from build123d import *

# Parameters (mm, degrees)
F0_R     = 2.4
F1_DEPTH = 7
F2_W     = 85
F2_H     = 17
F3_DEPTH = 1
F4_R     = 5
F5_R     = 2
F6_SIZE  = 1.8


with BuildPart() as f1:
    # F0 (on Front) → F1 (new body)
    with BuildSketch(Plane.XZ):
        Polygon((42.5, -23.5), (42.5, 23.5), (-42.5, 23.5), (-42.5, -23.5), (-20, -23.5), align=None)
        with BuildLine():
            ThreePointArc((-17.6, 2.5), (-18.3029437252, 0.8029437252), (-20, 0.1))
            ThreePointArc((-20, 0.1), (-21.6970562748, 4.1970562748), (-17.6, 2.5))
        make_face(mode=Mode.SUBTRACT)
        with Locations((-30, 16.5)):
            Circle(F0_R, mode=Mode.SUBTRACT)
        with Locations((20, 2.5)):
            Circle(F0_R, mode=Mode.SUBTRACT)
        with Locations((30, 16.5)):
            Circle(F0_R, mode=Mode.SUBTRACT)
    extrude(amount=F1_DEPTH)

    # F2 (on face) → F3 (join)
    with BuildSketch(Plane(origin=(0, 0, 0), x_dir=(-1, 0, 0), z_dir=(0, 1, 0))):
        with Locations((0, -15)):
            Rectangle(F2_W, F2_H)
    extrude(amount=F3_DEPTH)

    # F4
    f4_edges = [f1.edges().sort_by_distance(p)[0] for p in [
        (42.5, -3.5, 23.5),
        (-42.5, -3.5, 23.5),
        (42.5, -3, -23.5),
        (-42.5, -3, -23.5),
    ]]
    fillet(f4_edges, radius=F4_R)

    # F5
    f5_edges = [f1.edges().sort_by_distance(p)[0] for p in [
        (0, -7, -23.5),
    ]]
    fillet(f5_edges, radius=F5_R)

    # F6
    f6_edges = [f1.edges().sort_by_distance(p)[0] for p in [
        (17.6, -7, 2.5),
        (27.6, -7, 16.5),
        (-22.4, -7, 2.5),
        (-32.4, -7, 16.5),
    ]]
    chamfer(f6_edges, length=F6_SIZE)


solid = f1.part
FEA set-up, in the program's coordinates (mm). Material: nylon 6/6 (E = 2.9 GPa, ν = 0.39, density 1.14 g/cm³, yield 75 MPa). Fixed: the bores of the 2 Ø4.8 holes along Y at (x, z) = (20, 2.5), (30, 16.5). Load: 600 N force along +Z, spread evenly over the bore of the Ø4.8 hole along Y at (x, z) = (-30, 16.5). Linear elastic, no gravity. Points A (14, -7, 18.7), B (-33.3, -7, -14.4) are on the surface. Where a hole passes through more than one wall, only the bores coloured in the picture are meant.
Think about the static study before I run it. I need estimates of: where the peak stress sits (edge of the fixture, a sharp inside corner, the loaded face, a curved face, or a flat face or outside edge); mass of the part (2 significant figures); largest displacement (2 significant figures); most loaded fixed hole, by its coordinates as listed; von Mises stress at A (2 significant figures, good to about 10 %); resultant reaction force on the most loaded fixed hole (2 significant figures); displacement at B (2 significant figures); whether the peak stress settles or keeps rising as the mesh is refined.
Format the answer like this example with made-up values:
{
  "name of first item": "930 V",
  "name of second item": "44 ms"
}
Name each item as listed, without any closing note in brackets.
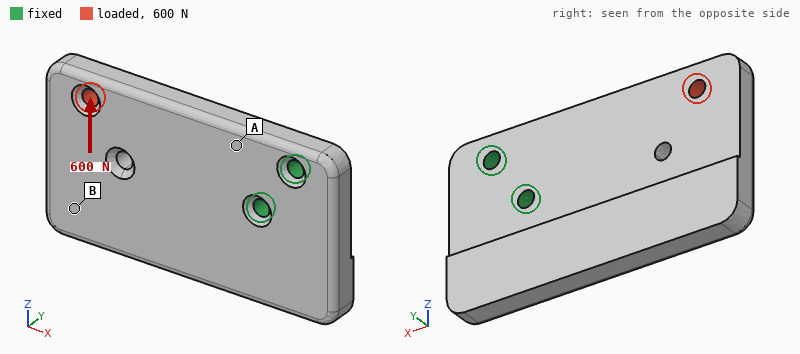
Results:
{
  "where the peak stress sits": "edge of the fixture",
  "mass of the part": "32 g",
  "largest displacement": "0.88 mm",
  "most loaded fixed hole, by its coordinates as listed": "(20, 2.5)",
  "von Mises stress at A": "11 MPa",
  "resultant reaction force on the most loaded fixed hole": "1.8 kN",
  "displacement at B": "0.73 mm",
  "whether the peak stress settles or keeps rising as the mesh is refined": "keeps rising"
}
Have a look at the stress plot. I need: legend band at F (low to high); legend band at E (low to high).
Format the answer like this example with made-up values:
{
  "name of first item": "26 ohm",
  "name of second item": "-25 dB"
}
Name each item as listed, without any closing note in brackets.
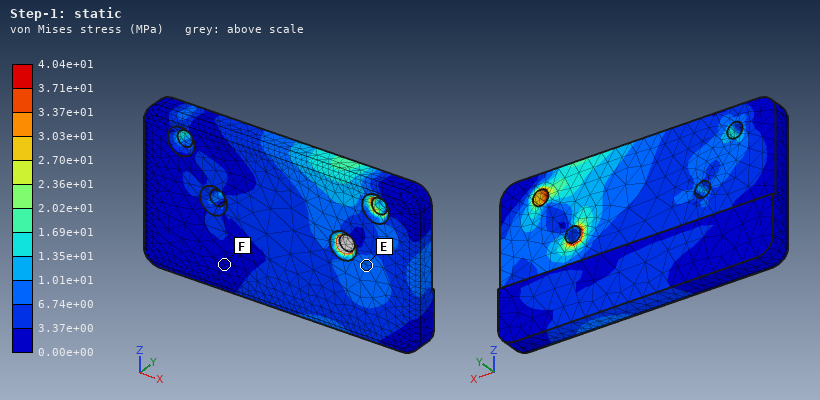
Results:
{
  "legend band at F": "0.00e+00 to 3.37e+00 MPa",
  "legend band at E": "6.74e+00 to 1.01e+01 MPa"
}
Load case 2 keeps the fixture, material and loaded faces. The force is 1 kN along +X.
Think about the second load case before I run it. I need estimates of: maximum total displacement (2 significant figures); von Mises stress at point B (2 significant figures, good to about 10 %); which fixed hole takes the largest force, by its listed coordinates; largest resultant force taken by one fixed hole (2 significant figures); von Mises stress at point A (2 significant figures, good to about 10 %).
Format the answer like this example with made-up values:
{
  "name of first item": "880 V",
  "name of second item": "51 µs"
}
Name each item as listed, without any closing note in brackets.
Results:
{
  "maximum total displacement": "0.63 mm",
  "von Mises stress at point B": "2.0 MPa",
  "which fixed hole takes the largest force, by its listed coordinates": "(30, 16.5)",
  "largest resultant force taken by one fixed hole": "790 N",
  "von Mises stress at point A": "6.0 MPa"
}
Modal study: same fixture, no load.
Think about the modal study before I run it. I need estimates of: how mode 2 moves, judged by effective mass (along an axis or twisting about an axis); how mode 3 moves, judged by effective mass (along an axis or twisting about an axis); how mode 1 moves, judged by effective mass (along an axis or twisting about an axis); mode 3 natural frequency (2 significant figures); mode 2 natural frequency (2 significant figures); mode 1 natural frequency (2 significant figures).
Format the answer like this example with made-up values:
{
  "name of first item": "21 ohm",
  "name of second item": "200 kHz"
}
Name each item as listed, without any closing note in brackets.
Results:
{
  "how mode 2 moves, judged by effective mass": "twisting about X",
  "how mode 3 moves, judged by effective mass": "along Z",
  "how mode 1 moves, judged by effective mass": "along Y",
  "mode 3 natural frequency": "1300 Hz",
  "mode 2 natural frequency": "1000 Hz",
  "mode 1 natural frequency": "410 Hz"
}
